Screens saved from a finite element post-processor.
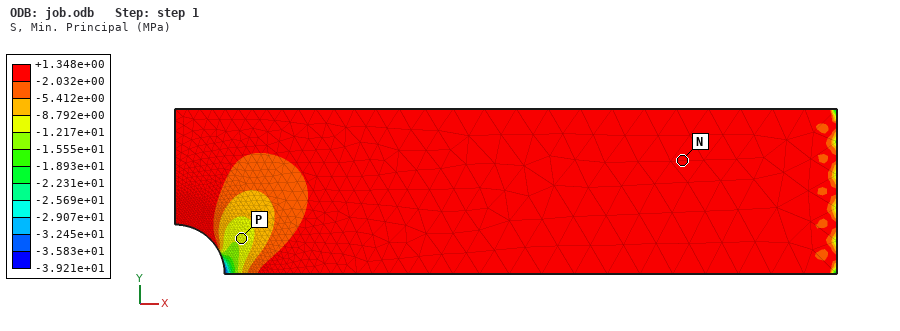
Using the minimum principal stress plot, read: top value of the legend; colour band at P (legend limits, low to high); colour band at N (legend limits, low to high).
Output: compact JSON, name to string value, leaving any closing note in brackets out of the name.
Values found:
{"top value of the legend": "+1.348e+00 MPa", "colour band at P": "-1.217e+01 to -8.792e+00 MPa", "colour band at N": "-2.032e+00 to +1.348e+00 MPa"}
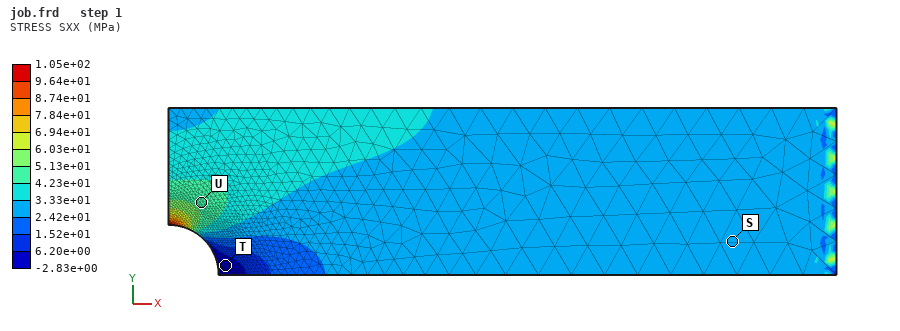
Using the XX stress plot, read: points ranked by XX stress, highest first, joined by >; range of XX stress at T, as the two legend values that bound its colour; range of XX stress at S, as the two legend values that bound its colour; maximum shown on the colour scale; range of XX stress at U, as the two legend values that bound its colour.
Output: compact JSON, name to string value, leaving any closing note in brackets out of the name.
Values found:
{"points ranked by XX stress, highest first, joined by >": "U > S > T", "range of XX stress at T, as the two legend values that bound its colour": "-2.83e+00 to 6.20e+00 MPa", "range of XX stress at S, as the two legend values that bound its colour": "2.42e+01 to 3.33e+01 MPa", "maximum shown on the colour scale": "1.05e+02 MPa", "range of XX stress at U, as the two legend values that bound its colour": "4.23e+01 to 5.13e+01 MPa"}
